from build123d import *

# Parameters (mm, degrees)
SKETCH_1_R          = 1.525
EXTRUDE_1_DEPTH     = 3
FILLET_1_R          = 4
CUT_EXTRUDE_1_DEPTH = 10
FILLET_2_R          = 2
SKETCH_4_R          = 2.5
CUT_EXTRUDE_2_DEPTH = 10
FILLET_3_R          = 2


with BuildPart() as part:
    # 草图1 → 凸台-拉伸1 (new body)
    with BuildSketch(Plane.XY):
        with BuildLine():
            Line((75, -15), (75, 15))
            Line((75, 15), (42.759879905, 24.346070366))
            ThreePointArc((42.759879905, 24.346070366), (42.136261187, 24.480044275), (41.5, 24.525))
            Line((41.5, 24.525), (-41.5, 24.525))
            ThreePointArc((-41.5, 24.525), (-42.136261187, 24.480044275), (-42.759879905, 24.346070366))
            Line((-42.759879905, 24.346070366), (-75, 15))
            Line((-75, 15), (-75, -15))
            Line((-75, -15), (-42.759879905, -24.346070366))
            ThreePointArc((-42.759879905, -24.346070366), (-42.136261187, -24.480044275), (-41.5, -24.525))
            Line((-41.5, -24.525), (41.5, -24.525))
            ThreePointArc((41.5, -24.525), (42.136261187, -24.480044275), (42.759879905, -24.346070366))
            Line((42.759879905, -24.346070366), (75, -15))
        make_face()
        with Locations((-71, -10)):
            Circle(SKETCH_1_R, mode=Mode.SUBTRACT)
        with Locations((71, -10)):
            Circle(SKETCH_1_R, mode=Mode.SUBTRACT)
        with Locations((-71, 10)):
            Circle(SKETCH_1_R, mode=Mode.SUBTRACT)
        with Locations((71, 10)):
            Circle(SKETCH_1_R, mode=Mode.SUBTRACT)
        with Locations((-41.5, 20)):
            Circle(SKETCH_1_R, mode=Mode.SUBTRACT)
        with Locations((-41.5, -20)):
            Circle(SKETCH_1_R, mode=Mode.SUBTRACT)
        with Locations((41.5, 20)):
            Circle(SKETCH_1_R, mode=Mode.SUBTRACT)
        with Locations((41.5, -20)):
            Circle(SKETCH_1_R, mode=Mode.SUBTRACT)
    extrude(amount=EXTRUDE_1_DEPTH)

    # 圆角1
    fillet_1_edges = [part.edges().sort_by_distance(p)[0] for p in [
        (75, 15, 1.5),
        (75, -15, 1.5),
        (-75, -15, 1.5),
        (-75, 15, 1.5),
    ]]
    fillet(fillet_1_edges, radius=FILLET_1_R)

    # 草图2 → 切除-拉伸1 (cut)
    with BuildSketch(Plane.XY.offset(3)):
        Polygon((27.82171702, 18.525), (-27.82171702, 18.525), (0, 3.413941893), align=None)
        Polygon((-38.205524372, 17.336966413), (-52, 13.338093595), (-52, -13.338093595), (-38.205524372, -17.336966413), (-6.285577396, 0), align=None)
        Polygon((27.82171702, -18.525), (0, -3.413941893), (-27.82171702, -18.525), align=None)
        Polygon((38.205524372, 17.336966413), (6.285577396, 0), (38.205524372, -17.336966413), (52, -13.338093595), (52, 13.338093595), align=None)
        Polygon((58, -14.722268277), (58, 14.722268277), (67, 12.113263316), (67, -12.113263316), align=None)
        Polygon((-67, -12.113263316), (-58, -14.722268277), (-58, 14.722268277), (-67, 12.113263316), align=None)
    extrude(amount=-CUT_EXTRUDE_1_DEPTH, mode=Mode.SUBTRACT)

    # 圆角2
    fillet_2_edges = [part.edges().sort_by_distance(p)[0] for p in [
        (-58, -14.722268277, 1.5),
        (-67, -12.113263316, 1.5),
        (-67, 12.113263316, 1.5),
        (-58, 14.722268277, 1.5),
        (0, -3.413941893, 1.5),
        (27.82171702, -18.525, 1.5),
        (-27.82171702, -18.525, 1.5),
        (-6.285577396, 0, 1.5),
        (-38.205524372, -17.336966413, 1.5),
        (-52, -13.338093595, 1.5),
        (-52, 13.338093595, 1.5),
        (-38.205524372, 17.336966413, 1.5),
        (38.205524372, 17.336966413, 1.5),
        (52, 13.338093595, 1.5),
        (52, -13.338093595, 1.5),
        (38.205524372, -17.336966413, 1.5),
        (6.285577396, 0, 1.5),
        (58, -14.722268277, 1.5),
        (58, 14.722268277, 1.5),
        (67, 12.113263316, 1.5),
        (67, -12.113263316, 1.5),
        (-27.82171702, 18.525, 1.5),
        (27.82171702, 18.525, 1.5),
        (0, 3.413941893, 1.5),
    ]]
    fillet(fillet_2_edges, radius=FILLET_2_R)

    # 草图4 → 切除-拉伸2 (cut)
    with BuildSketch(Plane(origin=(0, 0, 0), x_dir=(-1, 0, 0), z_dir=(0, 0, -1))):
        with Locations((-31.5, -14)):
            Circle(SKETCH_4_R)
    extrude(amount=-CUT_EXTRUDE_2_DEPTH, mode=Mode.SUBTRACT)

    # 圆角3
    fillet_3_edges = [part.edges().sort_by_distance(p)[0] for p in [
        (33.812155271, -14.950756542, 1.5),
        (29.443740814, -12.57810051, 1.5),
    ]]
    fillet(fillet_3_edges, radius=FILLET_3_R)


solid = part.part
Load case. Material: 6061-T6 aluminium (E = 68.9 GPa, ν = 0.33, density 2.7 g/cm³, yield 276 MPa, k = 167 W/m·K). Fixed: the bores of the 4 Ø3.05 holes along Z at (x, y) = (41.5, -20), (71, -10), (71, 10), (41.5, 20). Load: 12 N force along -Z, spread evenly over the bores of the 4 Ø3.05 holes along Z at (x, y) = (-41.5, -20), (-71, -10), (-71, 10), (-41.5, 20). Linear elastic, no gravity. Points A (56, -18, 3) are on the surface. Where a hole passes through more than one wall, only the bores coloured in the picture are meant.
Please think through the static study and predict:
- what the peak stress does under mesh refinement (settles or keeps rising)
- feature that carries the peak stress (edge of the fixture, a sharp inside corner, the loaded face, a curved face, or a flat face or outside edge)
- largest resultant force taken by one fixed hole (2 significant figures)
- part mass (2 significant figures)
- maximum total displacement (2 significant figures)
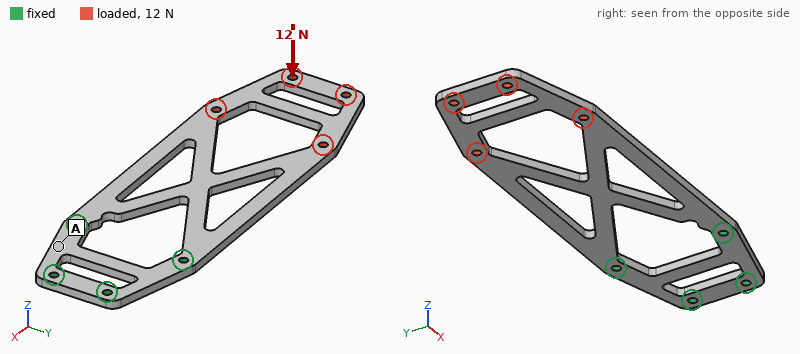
keeps rising
edge of the fixture
6.5 N
28 g
1.5 mm
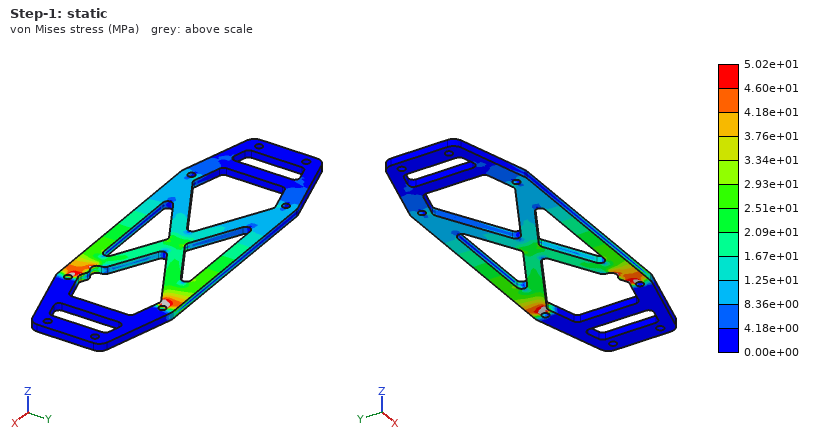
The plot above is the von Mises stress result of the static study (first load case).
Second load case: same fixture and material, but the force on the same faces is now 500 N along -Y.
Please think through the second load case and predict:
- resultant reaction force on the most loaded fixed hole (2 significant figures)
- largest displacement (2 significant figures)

1.1 kN
0.28 mm
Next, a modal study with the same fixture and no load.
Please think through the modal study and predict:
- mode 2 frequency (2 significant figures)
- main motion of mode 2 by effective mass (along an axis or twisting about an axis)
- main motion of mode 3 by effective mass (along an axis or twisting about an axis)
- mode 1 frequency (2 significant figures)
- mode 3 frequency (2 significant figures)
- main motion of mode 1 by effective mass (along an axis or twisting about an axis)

740 Hz
twisting about X
along Z
170 Hz
990 Hz
along Z
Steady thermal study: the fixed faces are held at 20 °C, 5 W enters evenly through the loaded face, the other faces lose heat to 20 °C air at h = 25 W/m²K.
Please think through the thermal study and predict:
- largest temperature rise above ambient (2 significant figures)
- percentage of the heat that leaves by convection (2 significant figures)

31 K
55 %
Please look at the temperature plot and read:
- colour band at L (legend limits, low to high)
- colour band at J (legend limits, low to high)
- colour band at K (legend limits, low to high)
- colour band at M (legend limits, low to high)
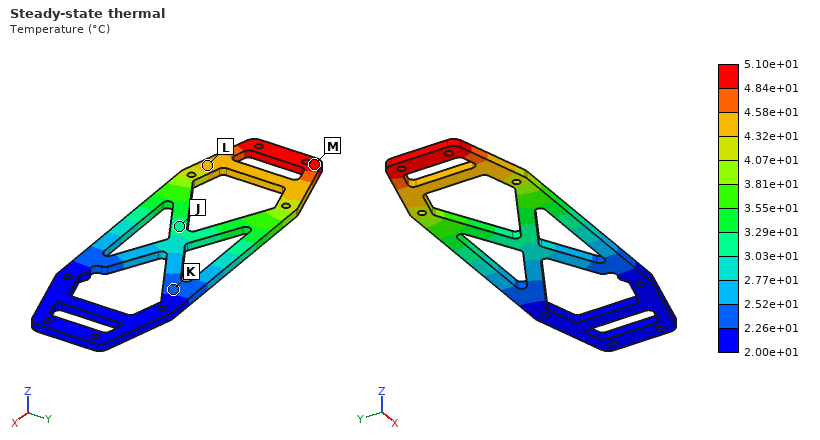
4.32e+01 to 4.58e+01 °C
3.03e+01 to 3.29e+01 °C
2.26e+01 to 2.52e+01 °C
4.84e+01 to 5.10e+01 °C
